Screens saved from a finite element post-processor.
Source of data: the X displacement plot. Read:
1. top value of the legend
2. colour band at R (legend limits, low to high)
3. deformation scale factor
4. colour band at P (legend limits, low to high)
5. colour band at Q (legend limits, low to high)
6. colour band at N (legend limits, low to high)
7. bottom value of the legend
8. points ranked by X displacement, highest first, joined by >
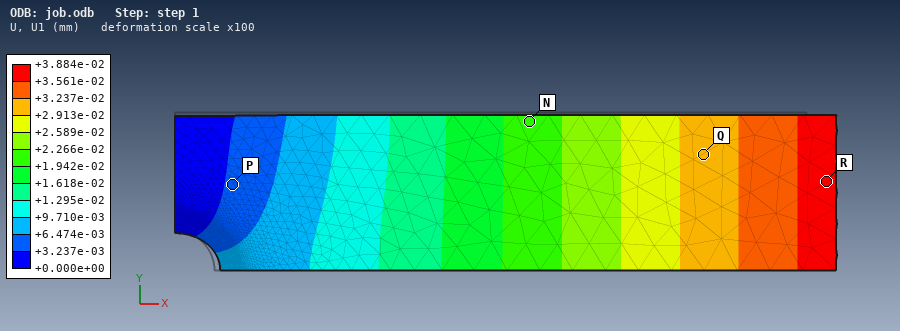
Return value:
+3.884e-02 mm
+3.561e-02 to +3.884e-02 mm
100
+3.237e-03 to +6.474e-03 mm
+2.913e-02 to +3.237e-02 mm
+1.942e-02 to +2.266e-02 mm
+0.000e+00 mm
R > Q > N > P
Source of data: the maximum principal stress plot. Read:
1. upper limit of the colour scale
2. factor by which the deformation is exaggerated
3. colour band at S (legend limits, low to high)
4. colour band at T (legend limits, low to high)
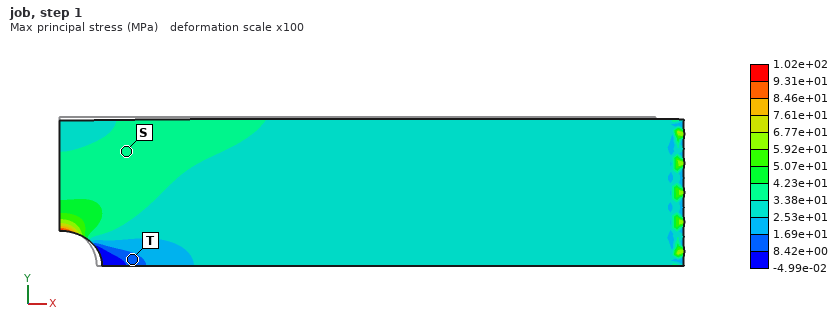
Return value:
1.02e+02 MPa
100
3.38e+01 to 4.23e+01 MPa
8.42e+00 to 1.69e+01 MPa
